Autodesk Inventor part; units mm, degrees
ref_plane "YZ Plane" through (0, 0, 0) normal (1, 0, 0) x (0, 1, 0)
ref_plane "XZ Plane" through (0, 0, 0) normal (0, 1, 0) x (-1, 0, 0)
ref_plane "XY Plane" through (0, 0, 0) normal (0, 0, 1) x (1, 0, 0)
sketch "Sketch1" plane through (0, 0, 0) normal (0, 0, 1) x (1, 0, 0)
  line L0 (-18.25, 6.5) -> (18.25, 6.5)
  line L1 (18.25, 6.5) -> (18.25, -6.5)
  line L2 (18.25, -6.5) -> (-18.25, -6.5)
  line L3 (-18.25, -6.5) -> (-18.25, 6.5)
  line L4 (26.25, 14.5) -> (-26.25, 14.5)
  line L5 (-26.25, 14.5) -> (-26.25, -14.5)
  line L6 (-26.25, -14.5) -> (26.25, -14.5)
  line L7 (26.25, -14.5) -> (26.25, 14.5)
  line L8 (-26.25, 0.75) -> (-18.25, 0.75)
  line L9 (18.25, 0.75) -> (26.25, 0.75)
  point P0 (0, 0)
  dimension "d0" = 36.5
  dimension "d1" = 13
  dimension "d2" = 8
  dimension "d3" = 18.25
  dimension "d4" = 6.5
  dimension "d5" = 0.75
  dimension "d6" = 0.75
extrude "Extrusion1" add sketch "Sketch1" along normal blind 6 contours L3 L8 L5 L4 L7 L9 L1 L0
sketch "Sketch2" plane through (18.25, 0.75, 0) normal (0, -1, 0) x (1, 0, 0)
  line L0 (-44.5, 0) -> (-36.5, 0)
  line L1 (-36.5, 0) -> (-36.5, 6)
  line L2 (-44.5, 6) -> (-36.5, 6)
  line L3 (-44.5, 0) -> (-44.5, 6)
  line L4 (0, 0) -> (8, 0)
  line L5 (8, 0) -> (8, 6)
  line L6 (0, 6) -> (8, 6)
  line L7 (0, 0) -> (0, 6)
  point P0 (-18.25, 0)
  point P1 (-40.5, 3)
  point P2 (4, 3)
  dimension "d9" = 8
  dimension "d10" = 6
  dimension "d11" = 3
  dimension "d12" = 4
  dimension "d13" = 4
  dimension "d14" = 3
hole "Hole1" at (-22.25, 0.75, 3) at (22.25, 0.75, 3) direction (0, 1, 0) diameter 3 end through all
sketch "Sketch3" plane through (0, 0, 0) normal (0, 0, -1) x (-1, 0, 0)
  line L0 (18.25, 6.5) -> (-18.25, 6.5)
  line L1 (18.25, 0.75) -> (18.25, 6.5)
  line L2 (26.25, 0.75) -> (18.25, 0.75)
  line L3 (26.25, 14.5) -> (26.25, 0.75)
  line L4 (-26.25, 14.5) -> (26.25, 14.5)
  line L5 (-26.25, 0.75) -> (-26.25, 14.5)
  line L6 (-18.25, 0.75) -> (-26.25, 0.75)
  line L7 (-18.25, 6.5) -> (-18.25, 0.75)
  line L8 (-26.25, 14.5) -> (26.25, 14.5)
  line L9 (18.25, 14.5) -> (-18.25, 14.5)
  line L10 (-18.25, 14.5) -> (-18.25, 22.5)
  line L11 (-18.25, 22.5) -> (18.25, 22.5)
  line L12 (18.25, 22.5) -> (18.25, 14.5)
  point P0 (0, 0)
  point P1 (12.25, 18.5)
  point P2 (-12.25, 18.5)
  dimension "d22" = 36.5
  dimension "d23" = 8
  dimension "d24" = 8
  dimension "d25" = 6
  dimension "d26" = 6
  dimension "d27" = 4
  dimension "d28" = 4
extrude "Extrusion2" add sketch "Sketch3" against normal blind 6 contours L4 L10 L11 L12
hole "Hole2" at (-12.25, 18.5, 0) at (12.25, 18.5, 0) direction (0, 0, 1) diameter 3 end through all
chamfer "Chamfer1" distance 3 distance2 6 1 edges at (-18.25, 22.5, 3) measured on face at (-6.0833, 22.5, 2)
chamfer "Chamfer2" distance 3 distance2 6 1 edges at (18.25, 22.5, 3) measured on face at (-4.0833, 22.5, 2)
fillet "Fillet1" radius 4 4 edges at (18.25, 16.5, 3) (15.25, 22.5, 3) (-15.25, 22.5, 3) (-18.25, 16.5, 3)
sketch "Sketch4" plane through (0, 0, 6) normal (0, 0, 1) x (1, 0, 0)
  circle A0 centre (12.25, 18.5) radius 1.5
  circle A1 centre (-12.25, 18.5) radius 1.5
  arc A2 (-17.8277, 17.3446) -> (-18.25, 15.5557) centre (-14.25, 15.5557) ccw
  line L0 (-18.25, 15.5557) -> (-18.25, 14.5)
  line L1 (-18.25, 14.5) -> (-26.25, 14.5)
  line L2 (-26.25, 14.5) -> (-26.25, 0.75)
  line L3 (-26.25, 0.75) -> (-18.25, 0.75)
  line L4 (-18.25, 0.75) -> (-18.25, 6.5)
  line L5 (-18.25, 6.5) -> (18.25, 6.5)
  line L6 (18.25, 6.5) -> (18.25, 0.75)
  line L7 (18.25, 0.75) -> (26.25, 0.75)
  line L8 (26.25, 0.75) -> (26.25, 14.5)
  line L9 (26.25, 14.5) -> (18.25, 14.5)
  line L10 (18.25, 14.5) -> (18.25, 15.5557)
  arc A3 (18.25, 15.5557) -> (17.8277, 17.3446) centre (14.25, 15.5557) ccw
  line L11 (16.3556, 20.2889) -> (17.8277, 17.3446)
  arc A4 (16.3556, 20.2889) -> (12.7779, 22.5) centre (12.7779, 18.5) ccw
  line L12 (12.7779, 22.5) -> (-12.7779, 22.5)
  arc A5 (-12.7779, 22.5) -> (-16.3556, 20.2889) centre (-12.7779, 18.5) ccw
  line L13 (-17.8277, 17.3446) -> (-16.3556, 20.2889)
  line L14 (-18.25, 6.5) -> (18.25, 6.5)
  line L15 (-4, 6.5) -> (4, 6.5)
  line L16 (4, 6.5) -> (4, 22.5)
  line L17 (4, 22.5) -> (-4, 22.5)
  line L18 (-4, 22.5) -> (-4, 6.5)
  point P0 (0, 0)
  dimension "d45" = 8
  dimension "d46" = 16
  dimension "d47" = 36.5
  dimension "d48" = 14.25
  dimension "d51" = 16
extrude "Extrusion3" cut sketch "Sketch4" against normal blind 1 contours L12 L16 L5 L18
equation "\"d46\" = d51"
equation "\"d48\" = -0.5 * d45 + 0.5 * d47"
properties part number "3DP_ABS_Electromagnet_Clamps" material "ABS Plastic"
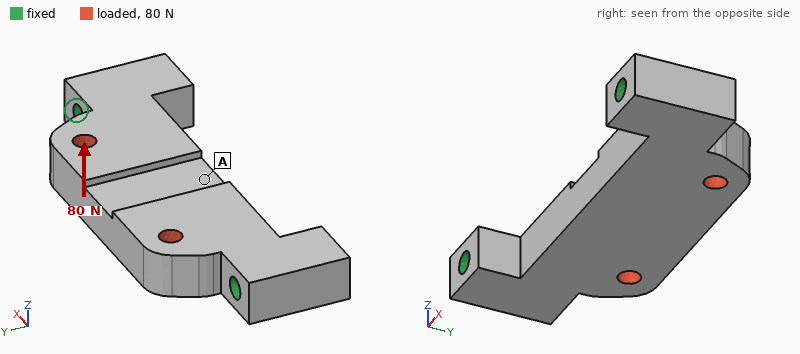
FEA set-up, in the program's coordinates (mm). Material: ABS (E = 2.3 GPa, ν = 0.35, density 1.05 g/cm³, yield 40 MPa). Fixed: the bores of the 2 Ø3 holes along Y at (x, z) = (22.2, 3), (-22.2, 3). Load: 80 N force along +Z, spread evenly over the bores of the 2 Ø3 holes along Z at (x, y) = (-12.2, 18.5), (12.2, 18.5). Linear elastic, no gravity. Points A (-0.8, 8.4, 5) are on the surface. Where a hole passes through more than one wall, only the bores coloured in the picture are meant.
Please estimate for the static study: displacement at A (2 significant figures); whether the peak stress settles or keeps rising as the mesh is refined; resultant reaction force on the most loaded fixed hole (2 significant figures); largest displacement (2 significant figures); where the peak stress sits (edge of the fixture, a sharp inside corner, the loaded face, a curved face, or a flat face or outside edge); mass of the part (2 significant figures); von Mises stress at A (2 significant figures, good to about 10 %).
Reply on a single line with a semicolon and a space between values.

0.033 mm; keeps rising; 40 N; 0.14 mm; edge of the fixture; 4.5 g; 1.4 MPa
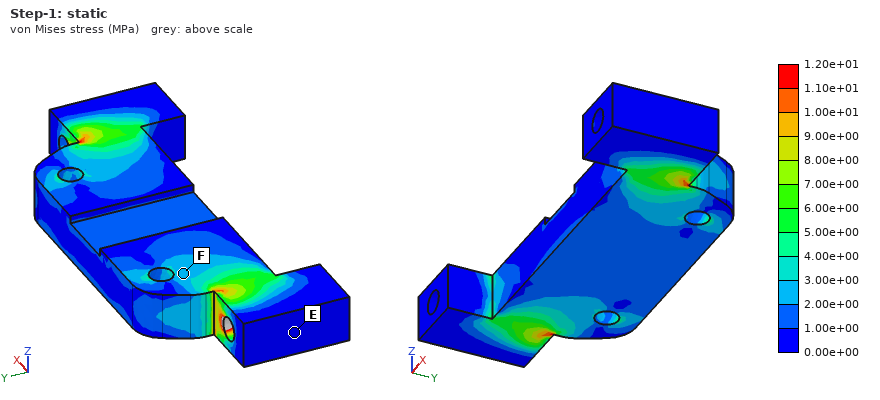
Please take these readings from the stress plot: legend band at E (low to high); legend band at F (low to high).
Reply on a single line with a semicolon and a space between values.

0.00e+00 to 1.00e+00 MPa; 2.00e+00 to 3.00e+00 MPa
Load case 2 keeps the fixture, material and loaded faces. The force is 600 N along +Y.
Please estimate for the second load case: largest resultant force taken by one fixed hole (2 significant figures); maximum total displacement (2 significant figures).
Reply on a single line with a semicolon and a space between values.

330 N; 98 µm
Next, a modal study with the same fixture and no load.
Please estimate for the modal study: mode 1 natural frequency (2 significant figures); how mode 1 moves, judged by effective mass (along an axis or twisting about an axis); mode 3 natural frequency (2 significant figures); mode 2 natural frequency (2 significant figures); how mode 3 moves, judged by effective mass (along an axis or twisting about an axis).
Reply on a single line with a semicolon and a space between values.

3000 Hz; along Z; 6600 Hz; 5600 Hz; along Y
